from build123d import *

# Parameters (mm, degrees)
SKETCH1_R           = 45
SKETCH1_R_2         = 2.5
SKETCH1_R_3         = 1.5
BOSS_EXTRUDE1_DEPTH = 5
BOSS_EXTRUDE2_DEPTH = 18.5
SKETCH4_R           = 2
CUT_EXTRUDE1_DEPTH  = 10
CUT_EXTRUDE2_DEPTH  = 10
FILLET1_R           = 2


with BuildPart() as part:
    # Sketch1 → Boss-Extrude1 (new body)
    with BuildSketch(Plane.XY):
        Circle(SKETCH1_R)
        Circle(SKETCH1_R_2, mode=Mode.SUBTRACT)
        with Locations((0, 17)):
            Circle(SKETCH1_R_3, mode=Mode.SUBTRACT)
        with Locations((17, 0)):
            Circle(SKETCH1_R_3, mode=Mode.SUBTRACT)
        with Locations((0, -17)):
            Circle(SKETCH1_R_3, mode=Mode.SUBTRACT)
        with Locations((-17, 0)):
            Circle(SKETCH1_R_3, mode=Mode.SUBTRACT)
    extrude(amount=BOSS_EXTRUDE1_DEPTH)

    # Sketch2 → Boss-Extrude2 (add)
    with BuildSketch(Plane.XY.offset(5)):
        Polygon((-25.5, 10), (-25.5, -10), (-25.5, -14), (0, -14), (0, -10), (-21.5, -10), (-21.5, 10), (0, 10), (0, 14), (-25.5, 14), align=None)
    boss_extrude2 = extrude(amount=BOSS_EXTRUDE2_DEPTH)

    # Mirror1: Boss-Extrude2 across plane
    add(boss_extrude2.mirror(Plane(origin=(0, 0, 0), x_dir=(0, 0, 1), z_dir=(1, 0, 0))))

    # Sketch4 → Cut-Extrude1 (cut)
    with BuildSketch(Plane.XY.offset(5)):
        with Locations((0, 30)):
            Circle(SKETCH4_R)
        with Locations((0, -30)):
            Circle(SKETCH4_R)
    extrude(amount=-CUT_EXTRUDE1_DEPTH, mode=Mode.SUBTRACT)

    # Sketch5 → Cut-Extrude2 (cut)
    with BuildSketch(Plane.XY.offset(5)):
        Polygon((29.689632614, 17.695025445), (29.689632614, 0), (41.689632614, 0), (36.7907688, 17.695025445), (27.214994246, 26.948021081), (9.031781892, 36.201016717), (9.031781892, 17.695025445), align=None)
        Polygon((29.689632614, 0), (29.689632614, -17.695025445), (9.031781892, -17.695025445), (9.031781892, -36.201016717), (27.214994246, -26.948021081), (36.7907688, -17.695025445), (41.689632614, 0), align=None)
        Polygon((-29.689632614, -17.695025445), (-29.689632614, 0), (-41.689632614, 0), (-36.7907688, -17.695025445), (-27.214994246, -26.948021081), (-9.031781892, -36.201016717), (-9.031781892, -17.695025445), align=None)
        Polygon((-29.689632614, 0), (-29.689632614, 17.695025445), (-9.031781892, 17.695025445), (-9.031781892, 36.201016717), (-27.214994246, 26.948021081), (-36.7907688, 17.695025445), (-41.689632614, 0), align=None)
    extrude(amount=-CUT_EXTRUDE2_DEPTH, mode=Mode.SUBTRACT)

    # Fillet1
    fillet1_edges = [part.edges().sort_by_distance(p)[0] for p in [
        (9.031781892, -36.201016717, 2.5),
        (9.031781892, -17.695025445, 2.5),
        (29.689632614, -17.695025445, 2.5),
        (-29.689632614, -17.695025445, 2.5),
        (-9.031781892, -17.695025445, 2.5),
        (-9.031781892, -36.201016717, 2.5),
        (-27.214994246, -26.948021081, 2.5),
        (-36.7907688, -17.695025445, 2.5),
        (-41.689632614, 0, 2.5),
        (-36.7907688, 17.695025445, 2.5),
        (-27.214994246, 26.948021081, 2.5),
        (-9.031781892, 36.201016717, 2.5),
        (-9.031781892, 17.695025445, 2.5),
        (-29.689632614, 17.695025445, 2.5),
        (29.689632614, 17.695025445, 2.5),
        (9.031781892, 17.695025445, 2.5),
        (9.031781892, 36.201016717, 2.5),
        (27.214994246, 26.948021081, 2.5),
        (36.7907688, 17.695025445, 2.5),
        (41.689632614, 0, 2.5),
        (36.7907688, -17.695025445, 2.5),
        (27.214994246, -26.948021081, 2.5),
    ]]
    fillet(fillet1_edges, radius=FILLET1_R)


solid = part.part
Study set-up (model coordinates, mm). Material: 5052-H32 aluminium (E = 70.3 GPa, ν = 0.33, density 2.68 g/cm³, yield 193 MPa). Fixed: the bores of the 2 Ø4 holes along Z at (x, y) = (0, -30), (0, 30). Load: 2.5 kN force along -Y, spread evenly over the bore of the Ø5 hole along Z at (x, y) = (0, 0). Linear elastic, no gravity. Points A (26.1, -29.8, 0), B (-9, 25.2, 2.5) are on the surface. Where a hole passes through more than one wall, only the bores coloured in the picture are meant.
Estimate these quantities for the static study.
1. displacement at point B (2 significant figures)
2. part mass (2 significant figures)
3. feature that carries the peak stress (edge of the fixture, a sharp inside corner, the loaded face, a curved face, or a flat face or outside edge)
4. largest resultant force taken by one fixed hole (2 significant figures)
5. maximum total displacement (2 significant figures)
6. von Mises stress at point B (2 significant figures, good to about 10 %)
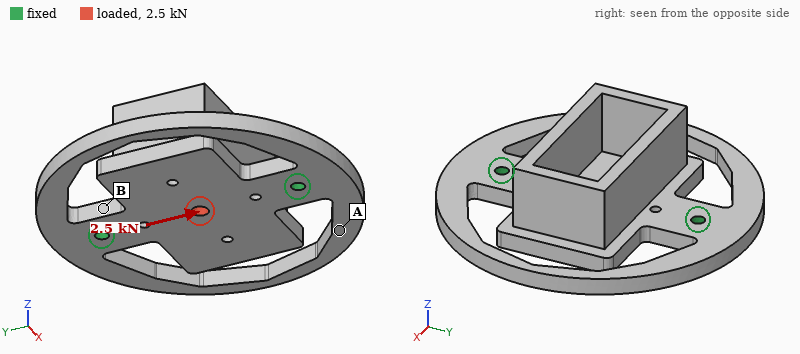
2.2 µm
88 g
the loaded face
1.3 kN
7.5 µm
8.8 MPa
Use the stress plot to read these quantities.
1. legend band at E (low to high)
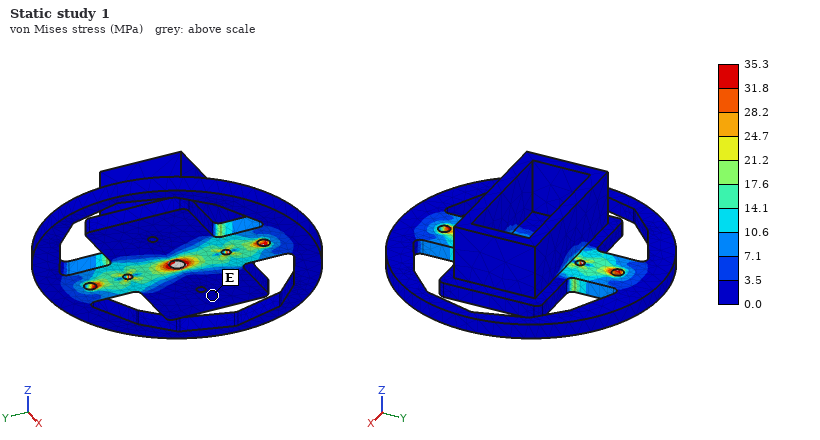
0.0 to 3.5 MPa
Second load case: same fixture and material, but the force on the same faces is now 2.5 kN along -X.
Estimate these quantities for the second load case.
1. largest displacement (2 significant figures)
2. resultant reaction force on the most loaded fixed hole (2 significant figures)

21 µm
1.3 kN
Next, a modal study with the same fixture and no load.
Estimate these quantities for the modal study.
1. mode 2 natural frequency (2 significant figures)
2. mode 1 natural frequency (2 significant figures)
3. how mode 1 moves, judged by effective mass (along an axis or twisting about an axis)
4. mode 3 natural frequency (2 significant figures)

1700 Hz
1600 Hz
twisting about Y
1700 Hz
